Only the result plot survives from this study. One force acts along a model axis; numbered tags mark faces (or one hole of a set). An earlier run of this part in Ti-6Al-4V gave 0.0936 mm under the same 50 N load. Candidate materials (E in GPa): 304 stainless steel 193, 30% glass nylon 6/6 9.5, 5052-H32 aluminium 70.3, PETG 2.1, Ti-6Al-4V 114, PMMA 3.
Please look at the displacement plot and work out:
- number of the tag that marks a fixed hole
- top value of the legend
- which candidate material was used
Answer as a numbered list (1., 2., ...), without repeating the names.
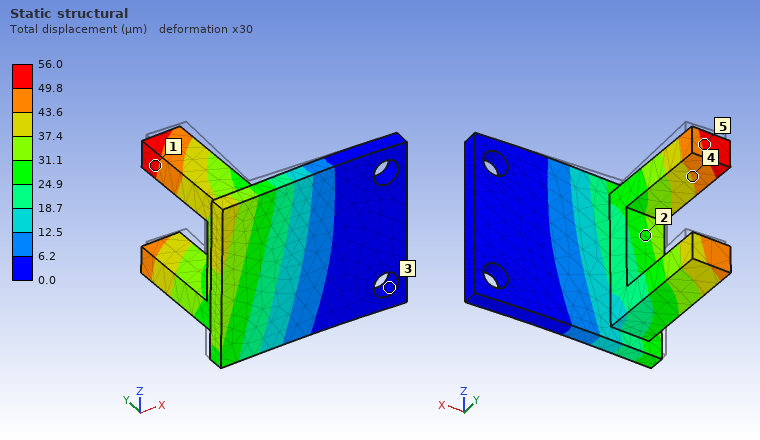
1. 3
2. 56.0 µm
3. 304 stainless steel
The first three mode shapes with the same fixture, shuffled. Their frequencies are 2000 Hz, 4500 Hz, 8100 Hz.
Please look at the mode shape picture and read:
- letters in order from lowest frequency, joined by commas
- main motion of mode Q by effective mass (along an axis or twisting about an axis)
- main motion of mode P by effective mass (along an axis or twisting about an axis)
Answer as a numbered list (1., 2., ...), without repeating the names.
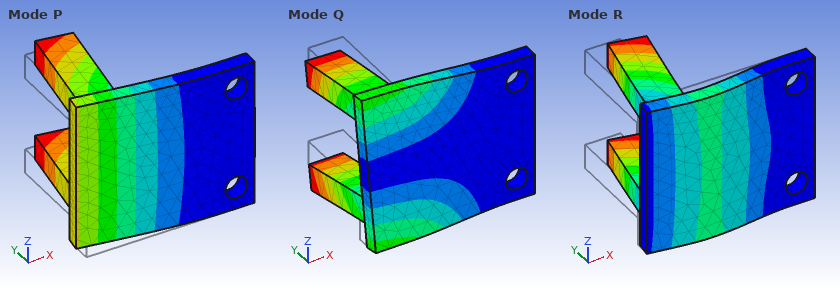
1. P, Q, R
2. along Z
3. along Y
